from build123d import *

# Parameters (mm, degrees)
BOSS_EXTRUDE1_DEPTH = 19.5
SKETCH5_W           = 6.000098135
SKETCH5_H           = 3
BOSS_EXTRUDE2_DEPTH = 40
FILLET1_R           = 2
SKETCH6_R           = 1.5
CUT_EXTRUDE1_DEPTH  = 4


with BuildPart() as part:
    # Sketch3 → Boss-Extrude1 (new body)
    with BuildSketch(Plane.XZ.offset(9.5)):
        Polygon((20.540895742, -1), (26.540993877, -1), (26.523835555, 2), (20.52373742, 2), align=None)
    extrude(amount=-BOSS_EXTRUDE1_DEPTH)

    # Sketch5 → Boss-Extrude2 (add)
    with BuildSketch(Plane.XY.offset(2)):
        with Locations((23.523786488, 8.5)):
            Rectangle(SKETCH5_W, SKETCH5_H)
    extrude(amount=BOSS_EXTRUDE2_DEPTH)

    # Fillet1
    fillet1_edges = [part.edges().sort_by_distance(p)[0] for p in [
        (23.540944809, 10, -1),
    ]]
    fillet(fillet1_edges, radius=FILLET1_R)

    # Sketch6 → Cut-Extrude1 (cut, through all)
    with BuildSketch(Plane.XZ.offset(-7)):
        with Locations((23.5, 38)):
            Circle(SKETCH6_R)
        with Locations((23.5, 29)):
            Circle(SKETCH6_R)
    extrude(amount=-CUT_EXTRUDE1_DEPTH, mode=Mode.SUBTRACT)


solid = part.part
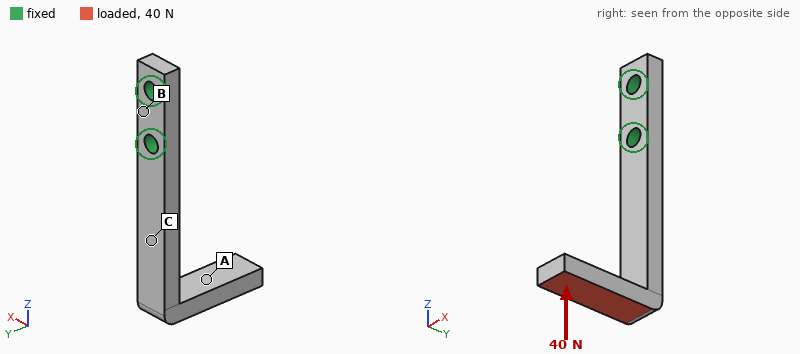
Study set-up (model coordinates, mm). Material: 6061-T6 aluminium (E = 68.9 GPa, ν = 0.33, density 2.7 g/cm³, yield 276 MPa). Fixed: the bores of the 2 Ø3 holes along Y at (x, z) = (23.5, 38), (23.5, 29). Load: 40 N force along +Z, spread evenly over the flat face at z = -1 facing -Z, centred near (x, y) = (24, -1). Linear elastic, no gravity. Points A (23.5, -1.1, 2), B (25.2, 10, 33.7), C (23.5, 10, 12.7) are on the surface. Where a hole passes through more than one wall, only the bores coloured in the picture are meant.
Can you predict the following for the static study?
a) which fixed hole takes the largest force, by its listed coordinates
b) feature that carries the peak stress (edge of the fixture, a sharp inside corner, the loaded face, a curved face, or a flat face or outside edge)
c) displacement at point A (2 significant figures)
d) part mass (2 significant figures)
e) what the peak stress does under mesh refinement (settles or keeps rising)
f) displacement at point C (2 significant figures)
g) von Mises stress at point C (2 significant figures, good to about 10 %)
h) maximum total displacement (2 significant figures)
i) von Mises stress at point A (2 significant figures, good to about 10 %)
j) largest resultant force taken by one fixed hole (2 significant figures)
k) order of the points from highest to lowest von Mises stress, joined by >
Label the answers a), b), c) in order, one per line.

a) (23.5, 29)
b) edge of the fixture
c) 0.17 mm
d) 2.8 g
e) keeps rising
f) 0.048 mm
g) 39 MPa
h) 0.28 mm
i) 9.2 MPa
j) 39 N
k) C > A > B
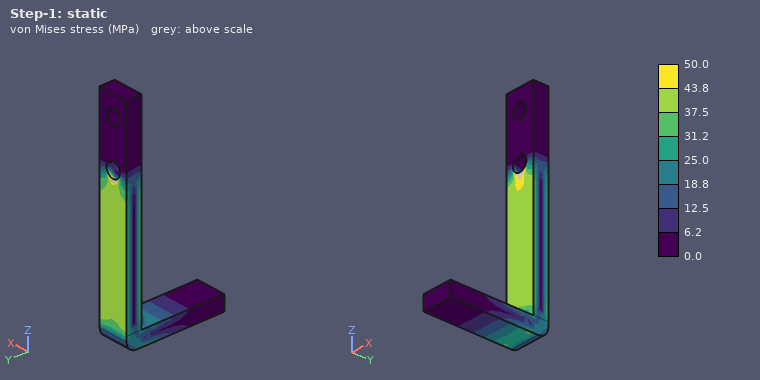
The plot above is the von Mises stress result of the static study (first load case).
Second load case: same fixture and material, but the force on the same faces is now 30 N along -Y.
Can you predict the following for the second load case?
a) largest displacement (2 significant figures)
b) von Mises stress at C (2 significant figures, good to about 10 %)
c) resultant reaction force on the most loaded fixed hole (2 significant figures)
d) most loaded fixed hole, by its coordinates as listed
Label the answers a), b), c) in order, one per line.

a) 0.36 mm
b) 46 MPa
c) 34 N
d) (23.5, 29)
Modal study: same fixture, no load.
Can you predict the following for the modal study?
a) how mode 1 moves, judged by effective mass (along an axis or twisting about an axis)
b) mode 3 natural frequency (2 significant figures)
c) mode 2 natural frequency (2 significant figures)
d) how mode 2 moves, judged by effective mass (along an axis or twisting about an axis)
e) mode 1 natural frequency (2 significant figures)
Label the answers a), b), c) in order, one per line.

a) along Y
b) 5100 Hz
c) 2300 Hz
d) along X
e) 1500 Hz
